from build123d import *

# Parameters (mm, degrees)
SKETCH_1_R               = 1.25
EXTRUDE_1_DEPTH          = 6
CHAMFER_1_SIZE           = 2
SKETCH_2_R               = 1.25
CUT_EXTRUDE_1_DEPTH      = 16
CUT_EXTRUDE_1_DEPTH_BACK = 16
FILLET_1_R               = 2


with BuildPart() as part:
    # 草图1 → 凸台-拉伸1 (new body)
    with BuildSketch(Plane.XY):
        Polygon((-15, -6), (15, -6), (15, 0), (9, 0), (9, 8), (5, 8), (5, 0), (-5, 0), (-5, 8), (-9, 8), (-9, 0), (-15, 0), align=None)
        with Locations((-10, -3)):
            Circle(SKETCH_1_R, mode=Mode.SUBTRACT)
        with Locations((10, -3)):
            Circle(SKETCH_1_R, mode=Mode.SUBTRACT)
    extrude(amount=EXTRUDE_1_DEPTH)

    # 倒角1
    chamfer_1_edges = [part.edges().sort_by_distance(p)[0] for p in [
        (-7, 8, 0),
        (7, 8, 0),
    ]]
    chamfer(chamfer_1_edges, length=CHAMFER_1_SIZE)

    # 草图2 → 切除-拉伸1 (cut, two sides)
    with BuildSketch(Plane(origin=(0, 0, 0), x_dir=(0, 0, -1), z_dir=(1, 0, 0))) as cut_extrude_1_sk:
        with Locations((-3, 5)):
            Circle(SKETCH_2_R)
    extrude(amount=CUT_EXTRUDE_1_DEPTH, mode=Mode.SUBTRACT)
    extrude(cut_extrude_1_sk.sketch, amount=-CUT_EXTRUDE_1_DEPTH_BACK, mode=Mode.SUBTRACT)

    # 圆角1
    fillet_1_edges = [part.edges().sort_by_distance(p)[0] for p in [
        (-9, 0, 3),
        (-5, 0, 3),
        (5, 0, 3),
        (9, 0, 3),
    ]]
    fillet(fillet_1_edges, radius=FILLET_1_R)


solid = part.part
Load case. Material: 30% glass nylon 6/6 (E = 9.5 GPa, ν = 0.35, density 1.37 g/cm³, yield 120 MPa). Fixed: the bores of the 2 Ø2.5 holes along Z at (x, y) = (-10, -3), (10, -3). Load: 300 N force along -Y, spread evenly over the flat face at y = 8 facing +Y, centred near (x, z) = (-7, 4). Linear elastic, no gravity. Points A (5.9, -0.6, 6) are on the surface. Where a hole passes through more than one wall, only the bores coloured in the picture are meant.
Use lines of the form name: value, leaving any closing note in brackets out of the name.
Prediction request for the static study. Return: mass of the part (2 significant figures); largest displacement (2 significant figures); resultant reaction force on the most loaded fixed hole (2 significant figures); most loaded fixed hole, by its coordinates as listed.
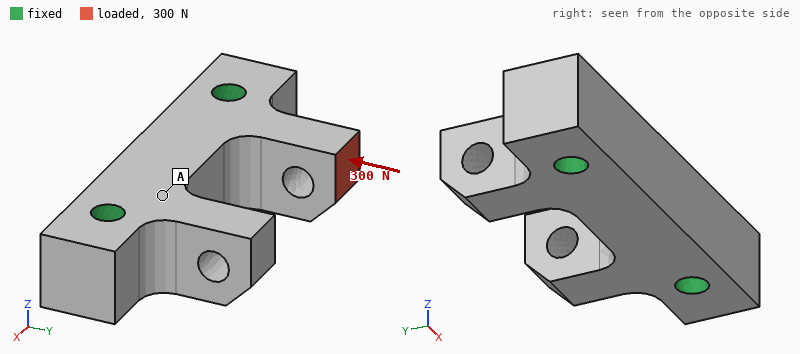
mass of the part: 1.9 g
largest displacement: 42 µm
resultant reaction force on the most loaded fixed hole: 270 N
most loaded fixed hole, by its coordinates as listed: (-10, -3)
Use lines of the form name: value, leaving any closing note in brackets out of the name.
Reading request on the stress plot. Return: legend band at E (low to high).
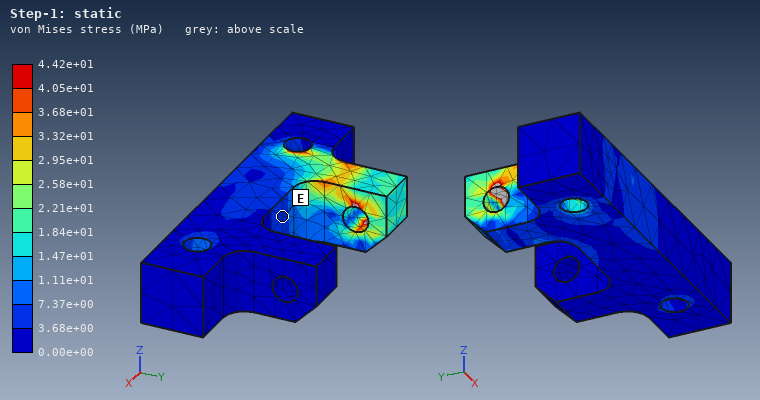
legend band at E: 3.68e+00 to 7.37e+00 MPa
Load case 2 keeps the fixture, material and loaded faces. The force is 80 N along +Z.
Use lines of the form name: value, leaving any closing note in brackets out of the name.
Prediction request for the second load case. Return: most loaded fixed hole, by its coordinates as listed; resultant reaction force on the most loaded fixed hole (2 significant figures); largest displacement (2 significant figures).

most loaded fixed hole, by its coordinates as listed: (-10, -3)
resultant reaction force on the most loaded fixed hole: 81 N
largest displacement: 69 µm
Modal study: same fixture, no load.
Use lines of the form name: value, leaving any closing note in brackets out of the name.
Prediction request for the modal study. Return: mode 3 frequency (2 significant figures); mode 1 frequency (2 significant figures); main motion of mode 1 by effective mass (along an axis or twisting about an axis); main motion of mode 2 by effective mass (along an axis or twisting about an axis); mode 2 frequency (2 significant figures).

mode 3 frequency: 21 kHz
mode 1 frequency: 17 kHz
main motion of mode 1 by effective mass: along Y
main motion of mode 2 by effective mass: along Z
mode 2 frequency: 19 kHz
